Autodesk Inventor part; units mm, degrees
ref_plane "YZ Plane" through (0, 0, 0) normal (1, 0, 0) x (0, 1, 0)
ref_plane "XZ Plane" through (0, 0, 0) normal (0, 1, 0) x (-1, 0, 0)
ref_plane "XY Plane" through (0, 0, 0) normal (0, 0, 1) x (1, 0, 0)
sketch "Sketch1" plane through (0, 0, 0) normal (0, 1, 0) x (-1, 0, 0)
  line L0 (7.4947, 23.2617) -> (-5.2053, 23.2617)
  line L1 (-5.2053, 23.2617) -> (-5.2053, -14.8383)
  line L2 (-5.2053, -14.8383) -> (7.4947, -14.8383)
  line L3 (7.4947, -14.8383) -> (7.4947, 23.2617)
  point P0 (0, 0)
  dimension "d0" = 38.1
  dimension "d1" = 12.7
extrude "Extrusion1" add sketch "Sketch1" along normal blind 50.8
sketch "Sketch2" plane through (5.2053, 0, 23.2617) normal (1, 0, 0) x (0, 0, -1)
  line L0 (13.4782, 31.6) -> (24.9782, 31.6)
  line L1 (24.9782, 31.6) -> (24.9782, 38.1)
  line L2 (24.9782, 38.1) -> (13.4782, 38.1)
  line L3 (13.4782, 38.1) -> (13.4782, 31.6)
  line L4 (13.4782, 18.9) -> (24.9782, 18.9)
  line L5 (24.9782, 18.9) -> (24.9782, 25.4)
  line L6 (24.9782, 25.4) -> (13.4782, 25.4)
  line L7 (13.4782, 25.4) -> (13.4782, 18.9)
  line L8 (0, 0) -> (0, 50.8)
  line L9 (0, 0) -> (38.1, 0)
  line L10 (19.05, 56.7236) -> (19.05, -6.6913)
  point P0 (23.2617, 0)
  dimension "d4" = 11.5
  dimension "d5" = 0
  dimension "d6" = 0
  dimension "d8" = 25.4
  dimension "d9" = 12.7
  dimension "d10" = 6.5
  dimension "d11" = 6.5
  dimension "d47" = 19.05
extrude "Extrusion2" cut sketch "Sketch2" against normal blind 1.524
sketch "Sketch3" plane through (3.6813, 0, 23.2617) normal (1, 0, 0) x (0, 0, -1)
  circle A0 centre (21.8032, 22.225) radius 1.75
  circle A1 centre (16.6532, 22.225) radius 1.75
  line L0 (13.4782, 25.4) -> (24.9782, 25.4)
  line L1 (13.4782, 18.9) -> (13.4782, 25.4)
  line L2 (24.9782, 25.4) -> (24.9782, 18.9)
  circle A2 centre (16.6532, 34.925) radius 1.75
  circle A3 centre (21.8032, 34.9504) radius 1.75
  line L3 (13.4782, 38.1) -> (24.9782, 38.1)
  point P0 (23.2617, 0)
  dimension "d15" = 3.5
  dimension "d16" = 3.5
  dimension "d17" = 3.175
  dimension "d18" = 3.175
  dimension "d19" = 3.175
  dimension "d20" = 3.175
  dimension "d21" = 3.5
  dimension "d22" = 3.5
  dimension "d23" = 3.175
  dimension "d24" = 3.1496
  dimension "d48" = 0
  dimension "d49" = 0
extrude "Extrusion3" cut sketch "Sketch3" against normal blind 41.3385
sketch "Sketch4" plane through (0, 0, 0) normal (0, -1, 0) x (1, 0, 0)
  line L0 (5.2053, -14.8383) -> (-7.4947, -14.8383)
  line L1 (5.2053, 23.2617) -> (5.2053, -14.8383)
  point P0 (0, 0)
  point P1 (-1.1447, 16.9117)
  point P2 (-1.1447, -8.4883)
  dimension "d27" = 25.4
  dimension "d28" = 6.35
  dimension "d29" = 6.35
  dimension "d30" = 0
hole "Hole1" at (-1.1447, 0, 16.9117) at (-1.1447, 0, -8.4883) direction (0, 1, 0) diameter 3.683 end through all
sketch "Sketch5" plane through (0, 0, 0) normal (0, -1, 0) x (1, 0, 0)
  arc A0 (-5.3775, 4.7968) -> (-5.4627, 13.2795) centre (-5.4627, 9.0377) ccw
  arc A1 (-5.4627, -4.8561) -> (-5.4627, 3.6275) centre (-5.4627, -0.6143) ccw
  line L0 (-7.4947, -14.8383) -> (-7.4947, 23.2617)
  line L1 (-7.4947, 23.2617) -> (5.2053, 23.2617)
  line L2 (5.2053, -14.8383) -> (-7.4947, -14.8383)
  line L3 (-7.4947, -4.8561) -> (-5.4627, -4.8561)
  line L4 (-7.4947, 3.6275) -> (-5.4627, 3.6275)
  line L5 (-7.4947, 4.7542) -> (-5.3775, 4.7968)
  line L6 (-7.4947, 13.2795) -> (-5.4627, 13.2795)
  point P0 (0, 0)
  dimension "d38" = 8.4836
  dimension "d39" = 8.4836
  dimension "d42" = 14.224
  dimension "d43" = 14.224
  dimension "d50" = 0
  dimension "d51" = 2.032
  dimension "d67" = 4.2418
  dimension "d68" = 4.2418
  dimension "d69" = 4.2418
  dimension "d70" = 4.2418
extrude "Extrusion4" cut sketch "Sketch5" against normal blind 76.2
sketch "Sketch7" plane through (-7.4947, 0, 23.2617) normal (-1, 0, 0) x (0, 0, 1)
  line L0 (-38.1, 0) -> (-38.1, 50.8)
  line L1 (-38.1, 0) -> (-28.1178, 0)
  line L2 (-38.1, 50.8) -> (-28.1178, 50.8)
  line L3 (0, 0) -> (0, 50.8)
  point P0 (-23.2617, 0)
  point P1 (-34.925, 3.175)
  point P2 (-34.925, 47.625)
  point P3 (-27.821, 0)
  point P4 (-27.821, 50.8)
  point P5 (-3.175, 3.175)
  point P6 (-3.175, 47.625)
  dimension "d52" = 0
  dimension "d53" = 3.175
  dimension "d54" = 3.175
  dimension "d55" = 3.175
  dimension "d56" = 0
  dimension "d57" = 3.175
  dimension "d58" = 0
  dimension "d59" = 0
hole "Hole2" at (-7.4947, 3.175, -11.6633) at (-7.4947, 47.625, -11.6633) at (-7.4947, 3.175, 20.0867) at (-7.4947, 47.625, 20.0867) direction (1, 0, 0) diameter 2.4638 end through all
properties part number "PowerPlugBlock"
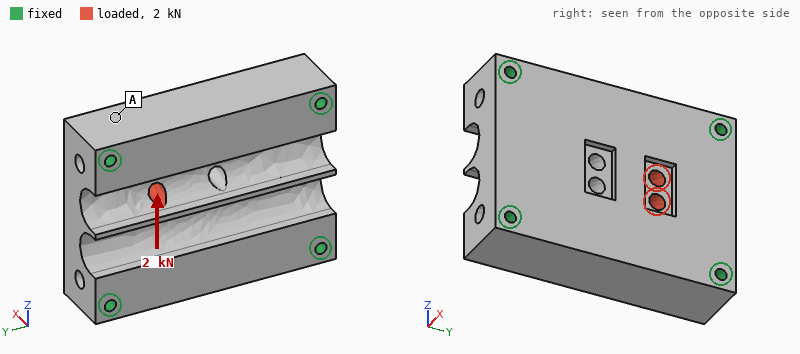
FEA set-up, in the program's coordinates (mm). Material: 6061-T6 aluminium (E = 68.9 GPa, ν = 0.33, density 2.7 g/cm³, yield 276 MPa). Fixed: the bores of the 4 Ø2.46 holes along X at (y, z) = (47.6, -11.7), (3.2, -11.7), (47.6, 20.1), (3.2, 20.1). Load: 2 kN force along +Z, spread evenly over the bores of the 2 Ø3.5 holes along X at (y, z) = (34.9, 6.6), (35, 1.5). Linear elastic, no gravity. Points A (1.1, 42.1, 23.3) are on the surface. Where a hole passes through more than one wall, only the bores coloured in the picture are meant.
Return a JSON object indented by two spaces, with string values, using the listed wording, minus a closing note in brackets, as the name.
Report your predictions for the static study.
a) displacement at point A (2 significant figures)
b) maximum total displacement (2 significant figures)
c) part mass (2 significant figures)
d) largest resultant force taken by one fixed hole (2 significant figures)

{
  "displacement at point A": "1.6 µm",
  "maximum total displacement": "7.4 µm",
  "part mass": "49 g",
  "largest resultant force taken by one fixed hole": "780 N"
}
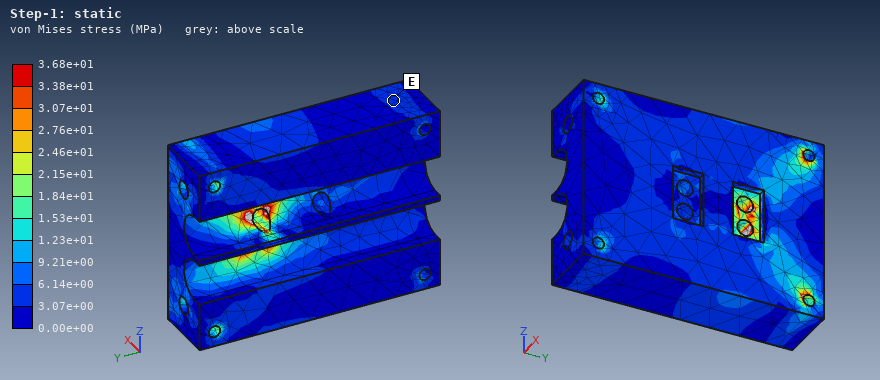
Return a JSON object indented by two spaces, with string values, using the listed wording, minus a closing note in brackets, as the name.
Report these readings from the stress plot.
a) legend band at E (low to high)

{
  "legend band at E": "3.07e+00 to 6.14e+00 MPa"
}
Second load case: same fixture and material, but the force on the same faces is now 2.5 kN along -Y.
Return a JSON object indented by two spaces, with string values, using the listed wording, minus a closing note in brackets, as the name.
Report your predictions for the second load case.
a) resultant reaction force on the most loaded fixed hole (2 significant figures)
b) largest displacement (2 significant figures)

{
  "resultant reaction force on the most loaded fixed hole": "810 N",
  "largest displacement": "5.2 µm"
}
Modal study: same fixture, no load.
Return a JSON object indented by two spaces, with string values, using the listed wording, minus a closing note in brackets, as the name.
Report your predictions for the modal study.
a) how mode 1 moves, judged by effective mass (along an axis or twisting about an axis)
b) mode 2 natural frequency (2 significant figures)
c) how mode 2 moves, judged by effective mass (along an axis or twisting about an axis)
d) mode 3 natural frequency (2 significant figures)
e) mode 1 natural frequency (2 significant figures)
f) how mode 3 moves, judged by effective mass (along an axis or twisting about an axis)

{
  "how mode 1 moves, judged by effective mass": "along X",
  "mode 2 natural frequency": "22 kHz",
  "how mode 2 moves, judged by effective mass": "along Z",
  "mode 3 natural frequency": "26 kHz",
  "mode 1 natural frequency": "17 kHz",
  "how mode 3 moves, judged by effective mass": "along Z"
}
